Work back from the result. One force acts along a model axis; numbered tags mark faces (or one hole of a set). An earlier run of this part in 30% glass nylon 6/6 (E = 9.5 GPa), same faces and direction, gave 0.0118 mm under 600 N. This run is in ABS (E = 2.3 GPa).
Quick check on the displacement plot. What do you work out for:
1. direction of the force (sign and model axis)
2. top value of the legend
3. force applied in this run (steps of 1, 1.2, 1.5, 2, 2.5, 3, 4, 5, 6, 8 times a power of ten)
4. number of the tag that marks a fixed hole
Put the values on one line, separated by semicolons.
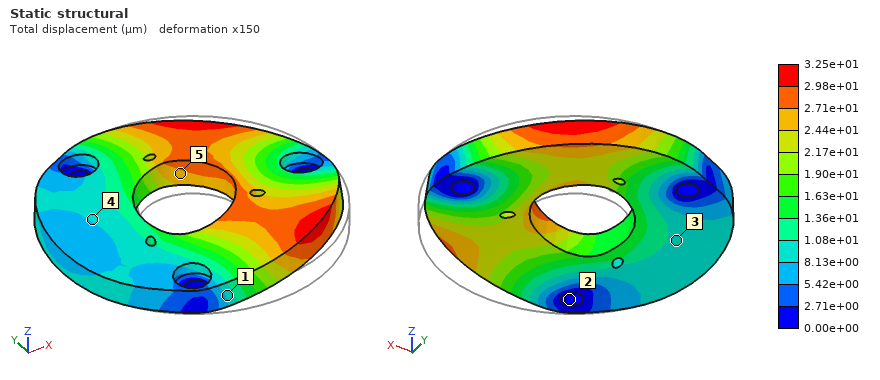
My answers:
+Y; 3.25e+01 µm; 400 N; 2
